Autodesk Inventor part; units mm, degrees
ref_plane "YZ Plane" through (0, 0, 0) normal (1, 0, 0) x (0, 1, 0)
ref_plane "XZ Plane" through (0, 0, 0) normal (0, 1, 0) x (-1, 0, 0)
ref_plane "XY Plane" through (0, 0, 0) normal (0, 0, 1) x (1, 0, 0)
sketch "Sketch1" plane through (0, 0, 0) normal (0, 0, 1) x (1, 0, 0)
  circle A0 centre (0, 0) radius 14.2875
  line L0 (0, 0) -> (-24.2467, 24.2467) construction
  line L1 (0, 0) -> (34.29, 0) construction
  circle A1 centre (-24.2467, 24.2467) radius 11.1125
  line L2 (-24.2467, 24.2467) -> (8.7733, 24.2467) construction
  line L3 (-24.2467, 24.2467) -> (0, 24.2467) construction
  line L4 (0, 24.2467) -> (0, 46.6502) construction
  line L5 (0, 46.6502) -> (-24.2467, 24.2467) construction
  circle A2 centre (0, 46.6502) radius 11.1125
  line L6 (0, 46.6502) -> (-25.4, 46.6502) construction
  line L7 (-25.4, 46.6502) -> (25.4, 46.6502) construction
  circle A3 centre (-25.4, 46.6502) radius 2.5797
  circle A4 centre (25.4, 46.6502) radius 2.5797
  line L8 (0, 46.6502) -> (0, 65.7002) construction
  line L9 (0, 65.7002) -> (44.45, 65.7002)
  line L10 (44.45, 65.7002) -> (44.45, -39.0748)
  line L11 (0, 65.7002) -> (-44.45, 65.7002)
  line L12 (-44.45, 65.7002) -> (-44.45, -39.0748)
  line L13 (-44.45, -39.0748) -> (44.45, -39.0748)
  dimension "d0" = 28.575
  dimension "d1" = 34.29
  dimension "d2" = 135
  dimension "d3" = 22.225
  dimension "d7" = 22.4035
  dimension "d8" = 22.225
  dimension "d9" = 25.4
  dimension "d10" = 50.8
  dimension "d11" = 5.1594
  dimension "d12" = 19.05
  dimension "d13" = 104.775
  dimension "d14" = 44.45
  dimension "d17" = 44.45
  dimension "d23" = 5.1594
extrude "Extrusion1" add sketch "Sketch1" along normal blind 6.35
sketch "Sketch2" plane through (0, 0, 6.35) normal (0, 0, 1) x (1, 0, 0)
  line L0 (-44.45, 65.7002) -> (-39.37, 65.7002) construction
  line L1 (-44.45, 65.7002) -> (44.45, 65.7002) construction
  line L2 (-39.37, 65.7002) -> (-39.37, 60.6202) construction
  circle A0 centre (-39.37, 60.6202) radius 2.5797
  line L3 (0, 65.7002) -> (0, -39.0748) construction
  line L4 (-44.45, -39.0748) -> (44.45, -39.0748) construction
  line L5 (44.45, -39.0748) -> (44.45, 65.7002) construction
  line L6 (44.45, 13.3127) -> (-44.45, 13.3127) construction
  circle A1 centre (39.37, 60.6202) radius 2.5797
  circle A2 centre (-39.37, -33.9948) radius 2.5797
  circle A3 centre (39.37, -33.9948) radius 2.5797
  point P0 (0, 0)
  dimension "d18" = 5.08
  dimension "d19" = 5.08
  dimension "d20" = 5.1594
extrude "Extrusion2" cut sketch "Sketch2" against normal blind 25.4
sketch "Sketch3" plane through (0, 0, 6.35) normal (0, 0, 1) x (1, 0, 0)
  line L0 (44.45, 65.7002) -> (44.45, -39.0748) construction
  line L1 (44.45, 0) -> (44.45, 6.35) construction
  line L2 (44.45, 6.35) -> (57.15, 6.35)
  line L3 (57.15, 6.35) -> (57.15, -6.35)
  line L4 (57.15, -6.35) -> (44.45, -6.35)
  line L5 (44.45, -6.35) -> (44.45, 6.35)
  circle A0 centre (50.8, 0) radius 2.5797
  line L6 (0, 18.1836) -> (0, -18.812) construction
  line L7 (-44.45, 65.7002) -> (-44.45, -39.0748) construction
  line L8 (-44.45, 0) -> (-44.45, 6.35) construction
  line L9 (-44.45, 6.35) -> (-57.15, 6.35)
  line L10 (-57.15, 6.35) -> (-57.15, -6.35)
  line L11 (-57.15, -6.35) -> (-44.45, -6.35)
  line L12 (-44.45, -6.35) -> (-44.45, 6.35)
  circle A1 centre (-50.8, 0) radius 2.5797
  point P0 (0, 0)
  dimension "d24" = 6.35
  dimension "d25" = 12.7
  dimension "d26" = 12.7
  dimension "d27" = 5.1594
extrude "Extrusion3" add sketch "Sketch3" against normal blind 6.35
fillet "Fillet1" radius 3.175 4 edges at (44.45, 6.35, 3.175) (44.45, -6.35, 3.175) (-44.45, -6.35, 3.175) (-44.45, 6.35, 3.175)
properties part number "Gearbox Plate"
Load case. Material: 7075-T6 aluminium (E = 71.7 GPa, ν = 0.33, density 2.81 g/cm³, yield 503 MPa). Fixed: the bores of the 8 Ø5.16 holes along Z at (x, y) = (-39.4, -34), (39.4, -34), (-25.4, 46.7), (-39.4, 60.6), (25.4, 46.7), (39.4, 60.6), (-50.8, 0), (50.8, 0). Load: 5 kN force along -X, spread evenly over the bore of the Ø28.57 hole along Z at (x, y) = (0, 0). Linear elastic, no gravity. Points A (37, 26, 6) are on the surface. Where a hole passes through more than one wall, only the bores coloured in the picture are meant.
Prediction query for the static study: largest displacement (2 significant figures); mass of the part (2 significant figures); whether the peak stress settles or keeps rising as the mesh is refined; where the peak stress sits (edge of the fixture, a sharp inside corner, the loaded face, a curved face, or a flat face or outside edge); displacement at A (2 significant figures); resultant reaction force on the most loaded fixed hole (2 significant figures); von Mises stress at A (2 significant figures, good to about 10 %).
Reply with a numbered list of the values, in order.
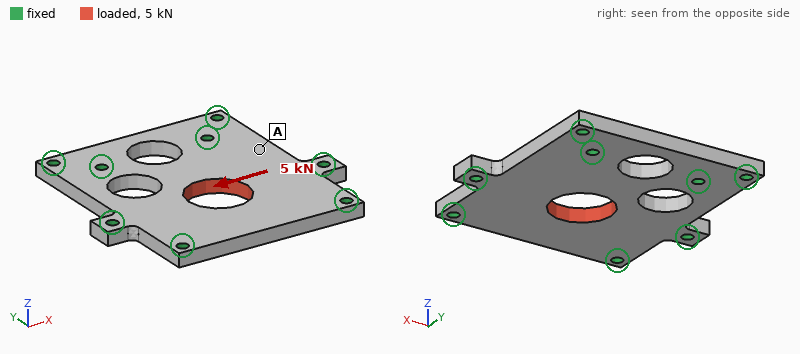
1. 7.0 µm
2. 140 g
3. keeps rising
4. edge of the fixture
5. 3.0 µm
6. 1.3 kN
7. 2.6 MPa
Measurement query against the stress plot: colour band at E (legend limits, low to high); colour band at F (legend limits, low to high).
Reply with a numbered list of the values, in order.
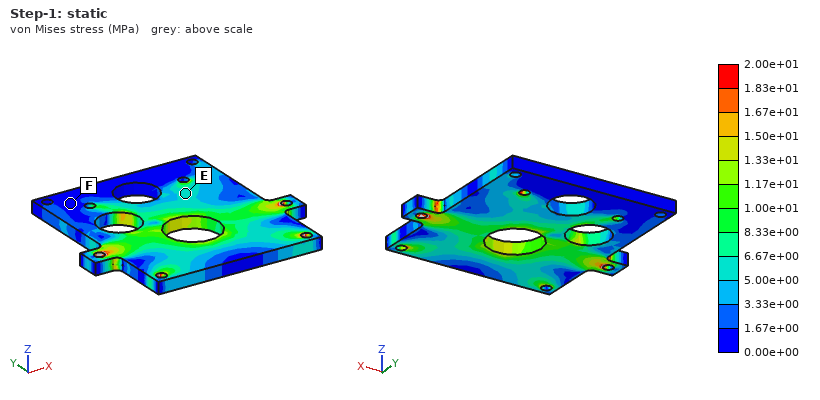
1. 5.00e+00 to 6.67e+00 MPa
2. 0.00e+00 to 1.67e+00 MPa
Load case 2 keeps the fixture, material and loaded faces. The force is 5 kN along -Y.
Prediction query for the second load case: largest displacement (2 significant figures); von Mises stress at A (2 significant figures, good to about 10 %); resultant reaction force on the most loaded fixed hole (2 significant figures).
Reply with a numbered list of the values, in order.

1. 10 µm
2. 3.3 MPa
3. 1.3 kN
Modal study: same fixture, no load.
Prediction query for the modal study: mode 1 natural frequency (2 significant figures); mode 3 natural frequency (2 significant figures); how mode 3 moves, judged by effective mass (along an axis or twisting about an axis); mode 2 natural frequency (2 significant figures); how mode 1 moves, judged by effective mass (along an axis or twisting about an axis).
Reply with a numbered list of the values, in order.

1. 4300 Hz
2. 8600 Hz
3. twisting about Y
4. 6700 Hz
5. along Z
